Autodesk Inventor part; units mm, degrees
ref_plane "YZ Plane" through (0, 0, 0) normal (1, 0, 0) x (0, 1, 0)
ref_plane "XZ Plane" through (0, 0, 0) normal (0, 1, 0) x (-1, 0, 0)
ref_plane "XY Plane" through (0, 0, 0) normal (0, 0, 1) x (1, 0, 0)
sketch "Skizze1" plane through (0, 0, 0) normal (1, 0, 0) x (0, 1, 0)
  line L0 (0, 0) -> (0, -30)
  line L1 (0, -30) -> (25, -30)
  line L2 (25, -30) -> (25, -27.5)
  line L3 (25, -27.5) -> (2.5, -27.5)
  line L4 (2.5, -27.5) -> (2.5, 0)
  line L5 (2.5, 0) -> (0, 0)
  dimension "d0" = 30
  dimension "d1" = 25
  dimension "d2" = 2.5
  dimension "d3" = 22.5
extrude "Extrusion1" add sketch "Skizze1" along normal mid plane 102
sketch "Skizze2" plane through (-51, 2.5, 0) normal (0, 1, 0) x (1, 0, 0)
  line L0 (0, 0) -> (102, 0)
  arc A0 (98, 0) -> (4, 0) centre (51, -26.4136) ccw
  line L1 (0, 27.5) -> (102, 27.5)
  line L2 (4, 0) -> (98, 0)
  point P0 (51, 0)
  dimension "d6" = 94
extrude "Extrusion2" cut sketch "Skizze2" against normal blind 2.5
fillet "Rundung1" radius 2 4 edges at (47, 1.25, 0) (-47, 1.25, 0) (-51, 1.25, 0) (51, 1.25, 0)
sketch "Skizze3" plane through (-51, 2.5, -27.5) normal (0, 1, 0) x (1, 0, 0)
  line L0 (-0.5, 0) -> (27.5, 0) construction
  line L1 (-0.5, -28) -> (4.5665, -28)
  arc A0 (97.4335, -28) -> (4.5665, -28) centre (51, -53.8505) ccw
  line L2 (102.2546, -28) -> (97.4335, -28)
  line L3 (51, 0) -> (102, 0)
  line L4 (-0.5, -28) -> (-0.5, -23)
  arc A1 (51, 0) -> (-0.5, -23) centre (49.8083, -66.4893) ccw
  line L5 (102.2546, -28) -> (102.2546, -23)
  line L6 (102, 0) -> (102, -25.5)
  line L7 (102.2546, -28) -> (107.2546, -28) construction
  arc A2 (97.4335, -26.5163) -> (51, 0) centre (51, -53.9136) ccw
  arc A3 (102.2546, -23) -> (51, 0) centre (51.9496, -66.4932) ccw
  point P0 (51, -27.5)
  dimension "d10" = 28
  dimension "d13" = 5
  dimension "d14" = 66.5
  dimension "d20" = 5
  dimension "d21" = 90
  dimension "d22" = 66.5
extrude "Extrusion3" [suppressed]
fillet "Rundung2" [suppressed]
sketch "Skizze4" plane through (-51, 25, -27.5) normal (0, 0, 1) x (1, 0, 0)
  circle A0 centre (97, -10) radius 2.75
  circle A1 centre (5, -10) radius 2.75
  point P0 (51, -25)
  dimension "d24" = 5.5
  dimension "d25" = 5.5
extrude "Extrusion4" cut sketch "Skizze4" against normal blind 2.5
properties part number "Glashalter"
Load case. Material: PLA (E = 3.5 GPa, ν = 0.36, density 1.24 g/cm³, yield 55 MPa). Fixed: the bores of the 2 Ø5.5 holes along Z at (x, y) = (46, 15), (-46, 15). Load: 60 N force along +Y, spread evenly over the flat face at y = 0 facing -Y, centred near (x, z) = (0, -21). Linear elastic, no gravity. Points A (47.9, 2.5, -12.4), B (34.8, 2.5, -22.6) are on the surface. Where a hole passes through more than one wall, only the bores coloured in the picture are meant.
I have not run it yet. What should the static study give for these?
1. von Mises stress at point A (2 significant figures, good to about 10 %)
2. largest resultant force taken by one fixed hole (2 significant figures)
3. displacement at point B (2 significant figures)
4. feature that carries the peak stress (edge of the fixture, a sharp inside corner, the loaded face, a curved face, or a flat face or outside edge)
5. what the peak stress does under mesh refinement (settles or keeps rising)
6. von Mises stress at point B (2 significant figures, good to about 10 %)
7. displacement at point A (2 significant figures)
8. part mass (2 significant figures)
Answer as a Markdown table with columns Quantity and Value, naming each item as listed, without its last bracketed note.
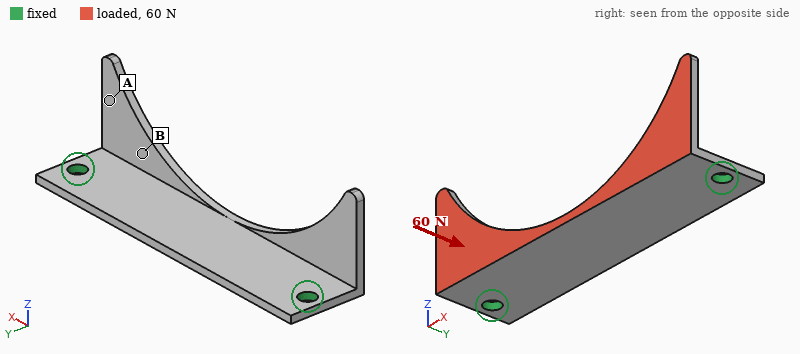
| Quantity | Value |
|---|---|
| von Mises stress at point A | 2.2 MPa |
| largest resultant force taken by one fixed hole | 30 N |
| displacement at point B | 0.24 mm |
| feature that carries the peak stress | edge of the fixture |
| what the peak stress does under mesh refinement | keeps rising |
| von Mises stress at point B | 5.0 MPa |
| displacement at point A | 0.61 mm |
| part mass | 11 g |
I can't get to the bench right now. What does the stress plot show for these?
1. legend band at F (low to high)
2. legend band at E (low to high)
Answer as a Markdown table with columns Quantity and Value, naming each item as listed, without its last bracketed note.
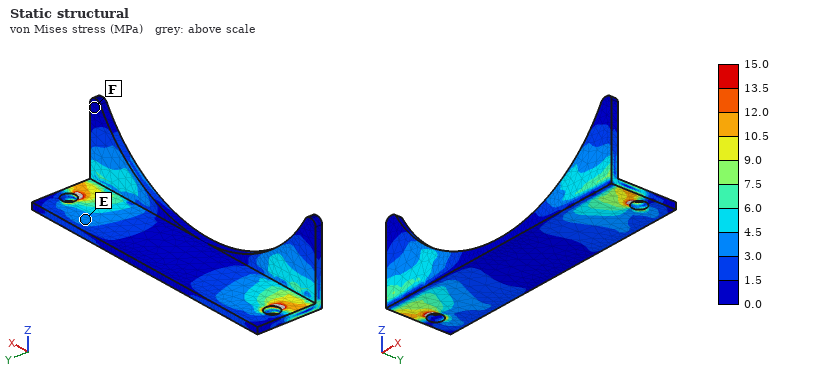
| Quantity | Value |
|---|---|
| legend band at F | 0.0 to 1.5 MPa |
| legend band at E | 3.0 to 4.5 MPa |
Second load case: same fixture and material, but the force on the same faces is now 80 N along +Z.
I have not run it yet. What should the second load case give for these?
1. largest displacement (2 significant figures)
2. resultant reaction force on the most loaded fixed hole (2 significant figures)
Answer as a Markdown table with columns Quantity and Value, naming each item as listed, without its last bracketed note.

| Quantity | Value |
|---|---|
| largest displacement | 1.3 mm |
| resultant reaction force on the most loaded fixed hole | 40 N |
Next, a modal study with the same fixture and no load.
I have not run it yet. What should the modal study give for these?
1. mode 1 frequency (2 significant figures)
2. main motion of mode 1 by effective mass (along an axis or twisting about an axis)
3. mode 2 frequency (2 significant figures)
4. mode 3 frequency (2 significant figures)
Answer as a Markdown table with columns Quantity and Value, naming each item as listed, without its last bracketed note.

| Quantity | Value |
|---|---|
| mode 1 frequency | 520 Hz |
| main motion of mode 1 by effective mass | along Z |
| mode 2 frequency | 720 Hz |
| mode 3 frequency | 820 Hz |
